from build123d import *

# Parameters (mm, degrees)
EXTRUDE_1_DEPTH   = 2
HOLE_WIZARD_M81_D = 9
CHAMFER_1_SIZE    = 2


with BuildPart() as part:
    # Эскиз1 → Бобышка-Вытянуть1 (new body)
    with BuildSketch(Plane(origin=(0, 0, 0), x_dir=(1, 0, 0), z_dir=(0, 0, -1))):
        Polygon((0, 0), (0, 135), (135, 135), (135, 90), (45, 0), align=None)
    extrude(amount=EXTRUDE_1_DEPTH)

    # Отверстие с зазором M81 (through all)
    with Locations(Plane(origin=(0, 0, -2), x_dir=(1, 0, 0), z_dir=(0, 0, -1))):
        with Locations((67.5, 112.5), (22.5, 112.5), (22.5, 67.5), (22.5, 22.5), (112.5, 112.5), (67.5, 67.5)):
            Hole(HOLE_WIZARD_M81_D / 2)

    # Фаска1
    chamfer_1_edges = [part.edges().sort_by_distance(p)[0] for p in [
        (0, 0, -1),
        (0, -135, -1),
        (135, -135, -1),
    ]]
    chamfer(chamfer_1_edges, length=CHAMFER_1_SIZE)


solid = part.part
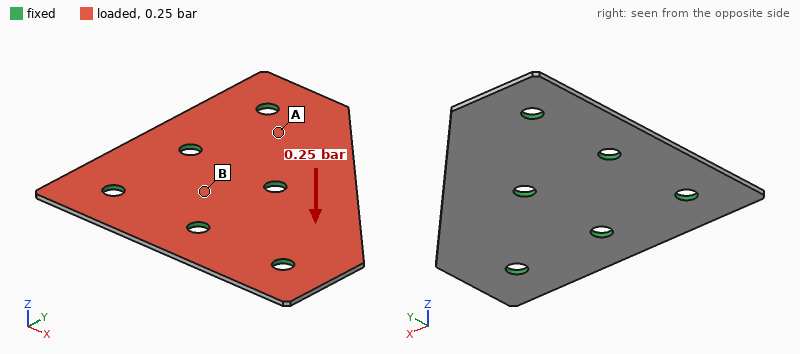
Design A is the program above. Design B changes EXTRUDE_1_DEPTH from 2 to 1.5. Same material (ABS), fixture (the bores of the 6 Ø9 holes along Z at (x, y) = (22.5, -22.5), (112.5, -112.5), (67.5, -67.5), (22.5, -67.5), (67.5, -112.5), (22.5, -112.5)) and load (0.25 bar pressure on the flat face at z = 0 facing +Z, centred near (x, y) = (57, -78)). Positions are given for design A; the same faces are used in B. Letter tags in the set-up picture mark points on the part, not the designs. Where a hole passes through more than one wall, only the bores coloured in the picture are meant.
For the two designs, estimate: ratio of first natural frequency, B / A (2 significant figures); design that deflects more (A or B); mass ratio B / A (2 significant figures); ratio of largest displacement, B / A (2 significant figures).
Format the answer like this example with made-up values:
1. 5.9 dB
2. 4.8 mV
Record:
1. 0.76
2. B
3. 0.75
4. 2.3
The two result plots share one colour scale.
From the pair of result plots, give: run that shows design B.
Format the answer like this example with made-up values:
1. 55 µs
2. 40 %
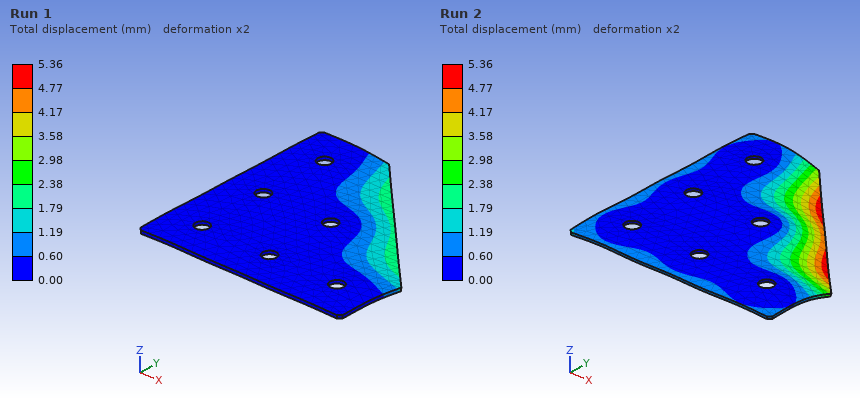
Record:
1. Run 2
